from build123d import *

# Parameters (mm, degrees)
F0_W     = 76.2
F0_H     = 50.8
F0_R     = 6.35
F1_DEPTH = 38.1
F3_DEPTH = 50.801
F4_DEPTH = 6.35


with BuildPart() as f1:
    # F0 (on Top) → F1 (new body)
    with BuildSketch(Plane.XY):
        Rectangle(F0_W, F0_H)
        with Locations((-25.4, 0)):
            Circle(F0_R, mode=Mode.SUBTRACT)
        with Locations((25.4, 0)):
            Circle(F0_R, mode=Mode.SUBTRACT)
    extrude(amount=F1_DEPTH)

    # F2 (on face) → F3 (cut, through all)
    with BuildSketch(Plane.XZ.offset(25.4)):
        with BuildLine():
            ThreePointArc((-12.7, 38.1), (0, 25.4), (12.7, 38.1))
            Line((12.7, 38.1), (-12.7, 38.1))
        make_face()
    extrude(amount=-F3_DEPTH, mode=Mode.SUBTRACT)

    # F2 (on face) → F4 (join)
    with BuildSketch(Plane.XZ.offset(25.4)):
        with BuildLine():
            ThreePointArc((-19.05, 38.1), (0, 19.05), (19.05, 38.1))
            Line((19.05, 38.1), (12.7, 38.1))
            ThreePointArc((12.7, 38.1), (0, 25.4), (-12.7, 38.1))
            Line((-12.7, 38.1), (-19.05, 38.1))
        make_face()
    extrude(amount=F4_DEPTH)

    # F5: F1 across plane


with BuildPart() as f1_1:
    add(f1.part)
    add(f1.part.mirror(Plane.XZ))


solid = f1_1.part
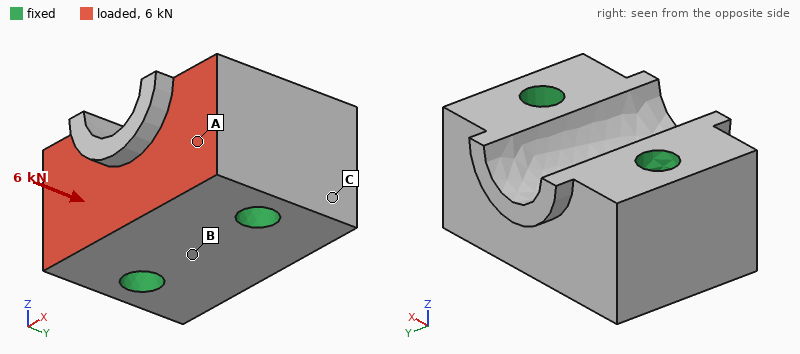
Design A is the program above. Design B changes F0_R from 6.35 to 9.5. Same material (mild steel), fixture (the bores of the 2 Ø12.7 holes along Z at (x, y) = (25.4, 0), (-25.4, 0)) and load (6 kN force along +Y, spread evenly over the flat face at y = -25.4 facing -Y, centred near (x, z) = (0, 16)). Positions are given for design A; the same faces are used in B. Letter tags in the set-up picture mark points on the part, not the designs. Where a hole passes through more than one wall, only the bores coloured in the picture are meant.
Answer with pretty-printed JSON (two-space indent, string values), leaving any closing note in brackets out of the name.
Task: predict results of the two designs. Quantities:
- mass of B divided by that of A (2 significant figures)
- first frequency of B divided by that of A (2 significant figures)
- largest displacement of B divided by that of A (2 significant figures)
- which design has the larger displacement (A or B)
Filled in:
{
  "mass of B divided by that of A": "0.91",
  "first frequency of B divided by that of A": "1.2",
  "largest displacement of B divided by that of A": "0.83",
  "which design has the larger displacement": "A"
}
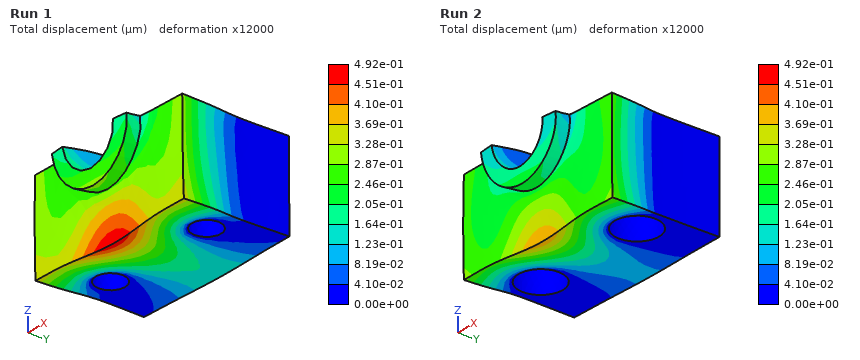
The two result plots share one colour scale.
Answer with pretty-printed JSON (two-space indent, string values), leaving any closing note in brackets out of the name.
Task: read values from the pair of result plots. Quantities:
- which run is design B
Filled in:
{
  "which run is design B": "Run 2"
}
